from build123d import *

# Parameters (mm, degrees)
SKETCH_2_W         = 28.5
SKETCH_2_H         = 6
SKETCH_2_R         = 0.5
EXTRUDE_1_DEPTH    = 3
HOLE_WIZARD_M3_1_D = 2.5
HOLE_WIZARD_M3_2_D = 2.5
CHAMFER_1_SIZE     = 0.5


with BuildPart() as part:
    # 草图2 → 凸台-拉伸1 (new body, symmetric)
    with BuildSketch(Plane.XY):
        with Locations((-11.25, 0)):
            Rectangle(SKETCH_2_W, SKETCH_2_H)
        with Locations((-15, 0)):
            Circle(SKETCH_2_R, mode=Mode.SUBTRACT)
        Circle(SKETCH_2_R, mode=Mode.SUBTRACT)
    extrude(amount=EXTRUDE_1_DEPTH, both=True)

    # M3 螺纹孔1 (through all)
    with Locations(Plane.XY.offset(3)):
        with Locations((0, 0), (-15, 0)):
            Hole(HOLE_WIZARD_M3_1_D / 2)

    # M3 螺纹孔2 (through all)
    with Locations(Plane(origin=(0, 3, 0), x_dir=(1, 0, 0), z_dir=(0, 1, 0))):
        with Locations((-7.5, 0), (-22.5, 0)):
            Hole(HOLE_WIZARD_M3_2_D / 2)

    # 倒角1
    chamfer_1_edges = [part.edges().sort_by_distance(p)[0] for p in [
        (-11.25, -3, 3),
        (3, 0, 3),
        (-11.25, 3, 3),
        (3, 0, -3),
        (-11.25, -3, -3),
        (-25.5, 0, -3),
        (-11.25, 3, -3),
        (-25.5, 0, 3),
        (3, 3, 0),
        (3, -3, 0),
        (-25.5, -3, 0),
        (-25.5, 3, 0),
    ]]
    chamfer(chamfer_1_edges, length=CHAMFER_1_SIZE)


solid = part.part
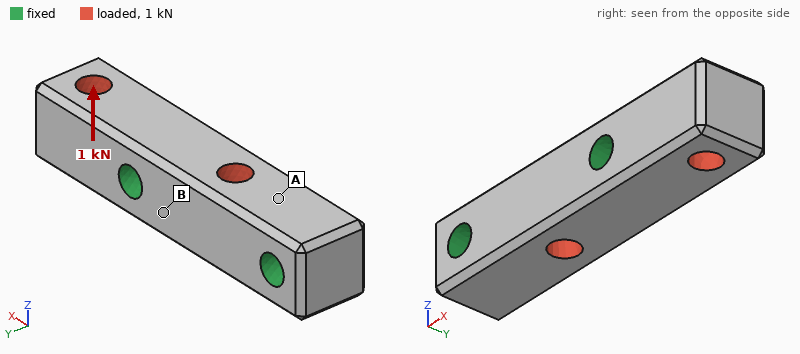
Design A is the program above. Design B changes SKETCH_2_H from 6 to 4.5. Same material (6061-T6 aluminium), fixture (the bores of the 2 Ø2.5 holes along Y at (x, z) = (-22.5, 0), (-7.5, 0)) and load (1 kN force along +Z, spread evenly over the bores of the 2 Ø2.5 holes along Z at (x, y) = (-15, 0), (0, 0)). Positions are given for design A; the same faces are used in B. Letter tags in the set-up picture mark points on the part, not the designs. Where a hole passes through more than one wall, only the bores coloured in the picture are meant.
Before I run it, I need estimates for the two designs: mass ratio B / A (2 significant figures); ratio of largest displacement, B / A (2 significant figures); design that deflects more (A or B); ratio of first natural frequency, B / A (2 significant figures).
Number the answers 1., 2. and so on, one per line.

1. 0.73
2. 1.4
3. B
4. 0.96
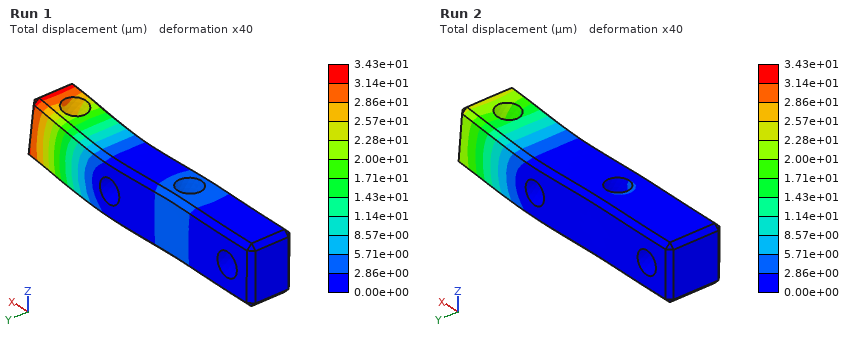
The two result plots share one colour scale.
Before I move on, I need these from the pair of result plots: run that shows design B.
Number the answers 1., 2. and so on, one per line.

1. Run 1
